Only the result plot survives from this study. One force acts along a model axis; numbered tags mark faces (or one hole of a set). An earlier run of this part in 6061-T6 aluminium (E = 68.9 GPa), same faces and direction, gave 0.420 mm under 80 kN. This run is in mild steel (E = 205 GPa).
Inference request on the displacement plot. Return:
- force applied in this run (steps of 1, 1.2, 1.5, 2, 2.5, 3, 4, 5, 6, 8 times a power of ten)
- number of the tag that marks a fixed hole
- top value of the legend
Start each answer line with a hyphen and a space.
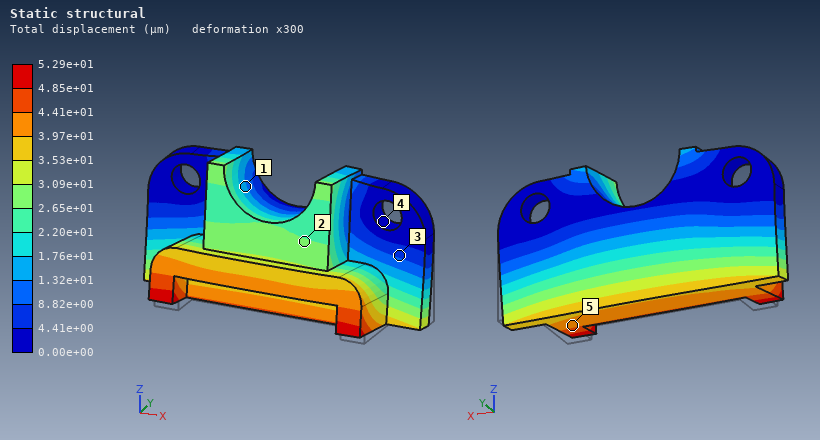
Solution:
- 30 kN
- 4
- 5.29e+01 µm
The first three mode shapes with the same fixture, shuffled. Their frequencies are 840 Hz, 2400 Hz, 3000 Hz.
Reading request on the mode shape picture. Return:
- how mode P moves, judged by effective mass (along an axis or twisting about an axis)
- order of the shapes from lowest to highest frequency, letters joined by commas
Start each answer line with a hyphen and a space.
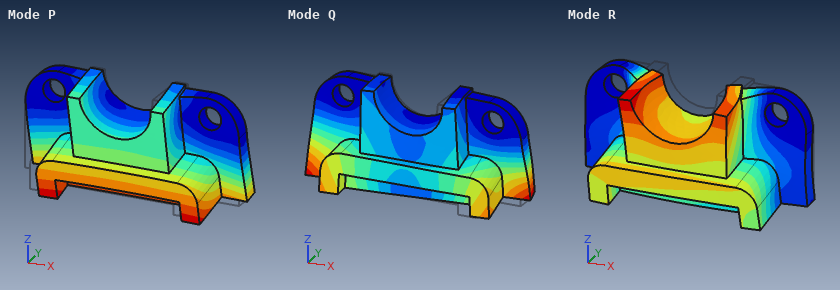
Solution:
- along Y
- P, Q, R
